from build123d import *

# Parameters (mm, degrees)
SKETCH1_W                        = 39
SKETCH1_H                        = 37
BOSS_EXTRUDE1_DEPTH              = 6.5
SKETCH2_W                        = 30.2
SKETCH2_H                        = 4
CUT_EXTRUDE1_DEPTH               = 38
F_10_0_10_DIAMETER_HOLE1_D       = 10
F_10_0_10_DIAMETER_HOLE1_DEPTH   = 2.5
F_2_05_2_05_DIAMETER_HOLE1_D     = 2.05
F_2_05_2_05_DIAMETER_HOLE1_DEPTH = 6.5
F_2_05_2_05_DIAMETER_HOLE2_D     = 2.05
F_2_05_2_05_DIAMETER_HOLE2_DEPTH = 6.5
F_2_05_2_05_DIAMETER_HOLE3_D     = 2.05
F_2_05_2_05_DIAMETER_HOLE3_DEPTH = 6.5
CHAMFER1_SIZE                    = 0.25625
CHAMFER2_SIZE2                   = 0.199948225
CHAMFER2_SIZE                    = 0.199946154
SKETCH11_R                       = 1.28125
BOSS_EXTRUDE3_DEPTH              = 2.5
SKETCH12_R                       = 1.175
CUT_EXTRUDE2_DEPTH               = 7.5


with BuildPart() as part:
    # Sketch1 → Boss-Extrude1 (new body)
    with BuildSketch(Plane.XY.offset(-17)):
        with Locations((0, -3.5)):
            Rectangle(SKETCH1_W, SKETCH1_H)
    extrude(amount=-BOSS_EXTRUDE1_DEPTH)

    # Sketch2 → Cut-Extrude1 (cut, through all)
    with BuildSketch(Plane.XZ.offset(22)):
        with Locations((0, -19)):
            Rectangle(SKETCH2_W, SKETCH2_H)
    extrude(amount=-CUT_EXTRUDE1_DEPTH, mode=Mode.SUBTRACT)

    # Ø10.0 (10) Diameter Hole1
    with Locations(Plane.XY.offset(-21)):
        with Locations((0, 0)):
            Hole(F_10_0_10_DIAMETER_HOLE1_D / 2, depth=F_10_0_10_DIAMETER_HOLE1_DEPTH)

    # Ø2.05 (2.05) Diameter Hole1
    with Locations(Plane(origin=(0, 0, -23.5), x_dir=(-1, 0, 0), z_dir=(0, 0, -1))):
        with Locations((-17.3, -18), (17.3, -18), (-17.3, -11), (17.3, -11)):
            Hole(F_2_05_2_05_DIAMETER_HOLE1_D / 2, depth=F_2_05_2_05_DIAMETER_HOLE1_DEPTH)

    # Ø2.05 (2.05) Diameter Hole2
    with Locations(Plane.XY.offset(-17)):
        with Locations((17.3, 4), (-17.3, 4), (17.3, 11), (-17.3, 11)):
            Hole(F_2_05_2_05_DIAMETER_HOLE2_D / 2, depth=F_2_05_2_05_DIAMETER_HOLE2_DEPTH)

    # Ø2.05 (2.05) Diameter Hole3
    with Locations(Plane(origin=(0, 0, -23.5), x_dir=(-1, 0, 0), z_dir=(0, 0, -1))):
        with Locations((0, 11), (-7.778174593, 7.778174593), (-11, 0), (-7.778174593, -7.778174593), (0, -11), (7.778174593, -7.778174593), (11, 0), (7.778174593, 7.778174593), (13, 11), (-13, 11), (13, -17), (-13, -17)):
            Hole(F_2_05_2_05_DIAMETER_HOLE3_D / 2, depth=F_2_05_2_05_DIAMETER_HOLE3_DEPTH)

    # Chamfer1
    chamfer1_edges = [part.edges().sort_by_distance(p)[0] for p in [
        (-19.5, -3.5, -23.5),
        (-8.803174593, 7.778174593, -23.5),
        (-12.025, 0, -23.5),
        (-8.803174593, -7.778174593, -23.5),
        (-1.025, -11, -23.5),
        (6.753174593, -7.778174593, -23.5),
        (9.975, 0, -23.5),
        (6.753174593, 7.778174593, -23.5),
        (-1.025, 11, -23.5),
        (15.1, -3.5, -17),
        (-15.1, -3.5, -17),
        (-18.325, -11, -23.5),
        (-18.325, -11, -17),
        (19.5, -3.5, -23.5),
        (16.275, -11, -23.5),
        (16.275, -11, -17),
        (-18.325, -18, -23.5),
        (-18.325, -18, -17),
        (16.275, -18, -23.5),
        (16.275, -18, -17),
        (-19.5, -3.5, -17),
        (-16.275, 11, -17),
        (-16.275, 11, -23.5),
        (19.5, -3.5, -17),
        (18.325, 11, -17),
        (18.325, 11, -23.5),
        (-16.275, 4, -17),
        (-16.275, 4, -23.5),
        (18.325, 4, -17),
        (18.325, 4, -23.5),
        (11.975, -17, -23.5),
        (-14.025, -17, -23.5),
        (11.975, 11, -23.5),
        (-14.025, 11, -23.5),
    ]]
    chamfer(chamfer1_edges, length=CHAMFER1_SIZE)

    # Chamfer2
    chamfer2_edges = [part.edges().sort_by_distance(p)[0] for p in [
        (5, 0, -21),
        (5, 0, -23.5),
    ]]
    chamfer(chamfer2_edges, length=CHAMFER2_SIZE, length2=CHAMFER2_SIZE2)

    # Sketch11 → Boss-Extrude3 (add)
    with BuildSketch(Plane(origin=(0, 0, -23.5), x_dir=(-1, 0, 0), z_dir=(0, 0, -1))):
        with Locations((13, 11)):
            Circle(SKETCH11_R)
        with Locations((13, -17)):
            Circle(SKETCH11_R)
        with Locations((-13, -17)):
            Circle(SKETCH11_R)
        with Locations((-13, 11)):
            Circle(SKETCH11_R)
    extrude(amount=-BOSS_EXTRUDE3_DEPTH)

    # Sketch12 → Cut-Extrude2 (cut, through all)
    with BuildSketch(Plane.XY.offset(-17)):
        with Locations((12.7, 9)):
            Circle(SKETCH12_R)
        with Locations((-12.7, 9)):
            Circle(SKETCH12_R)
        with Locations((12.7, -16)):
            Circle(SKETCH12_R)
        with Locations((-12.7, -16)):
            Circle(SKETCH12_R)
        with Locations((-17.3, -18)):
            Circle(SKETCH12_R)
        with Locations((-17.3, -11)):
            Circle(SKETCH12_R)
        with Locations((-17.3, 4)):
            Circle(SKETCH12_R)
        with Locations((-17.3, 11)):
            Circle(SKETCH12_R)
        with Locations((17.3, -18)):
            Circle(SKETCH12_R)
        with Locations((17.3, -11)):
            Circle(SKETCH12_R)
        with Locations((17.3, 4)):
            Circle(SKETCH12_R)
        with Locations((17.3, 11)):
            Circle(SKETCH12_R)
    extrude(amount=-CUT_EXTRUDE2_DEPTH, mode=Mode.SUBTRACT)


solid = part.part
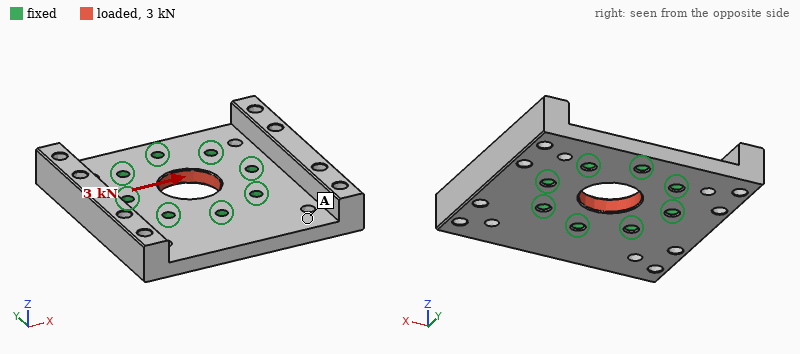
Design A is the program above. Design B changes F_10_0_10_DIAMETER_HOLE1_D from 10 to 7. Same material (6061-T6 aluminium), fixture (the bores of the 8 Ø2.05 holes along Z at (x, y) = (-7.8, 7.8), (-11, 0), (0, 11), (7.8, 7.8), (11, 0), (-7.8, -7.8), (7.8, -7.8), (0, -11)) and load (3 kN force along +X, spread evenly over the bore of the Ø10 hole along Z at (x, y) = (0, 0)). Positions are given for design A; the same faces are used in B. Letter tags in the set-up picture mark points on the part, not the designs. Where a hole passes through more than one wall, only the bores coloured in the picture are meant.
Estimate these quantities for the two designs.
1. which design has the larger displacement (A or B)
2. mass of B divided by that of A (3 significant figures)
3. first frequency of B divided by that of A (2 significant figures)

B
1.02
1.0
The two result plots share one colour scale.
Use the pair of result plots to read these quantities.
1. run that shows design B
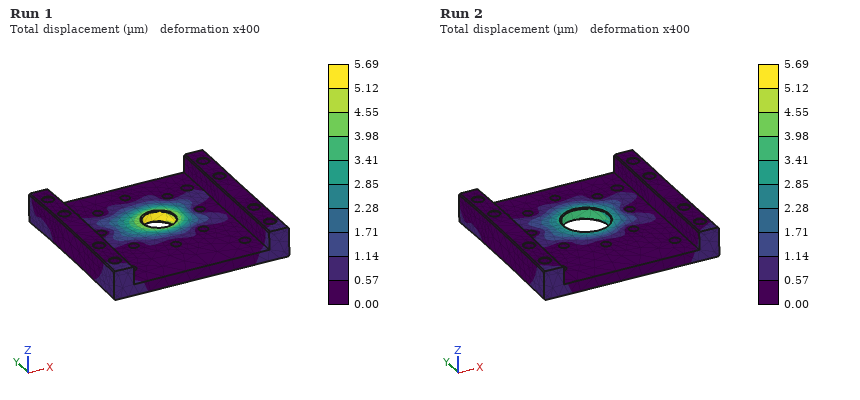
Run 1
